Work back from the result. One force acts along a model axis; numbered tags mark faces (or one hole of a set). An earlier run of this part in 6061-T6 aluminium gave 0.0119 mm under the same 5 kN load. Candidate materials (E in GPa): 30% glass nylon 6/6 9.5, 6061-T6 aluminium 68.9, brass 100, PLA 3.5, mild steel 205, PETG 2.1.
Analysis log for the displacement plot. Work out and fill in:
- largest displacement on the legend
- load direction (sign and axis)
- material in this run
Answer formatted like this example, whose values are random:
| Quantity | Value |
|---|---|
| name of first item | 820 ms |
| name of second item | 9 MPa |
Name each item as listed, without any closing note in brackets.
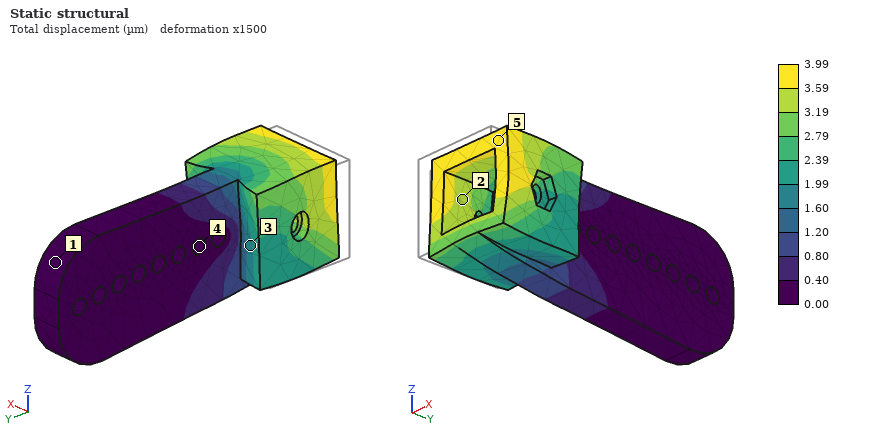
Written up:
| Quantity | Value |
|---|---|
| largest displacement on the legend | 3.99 µm |
| load direction | +Y |
| material in this run | mild steel |
